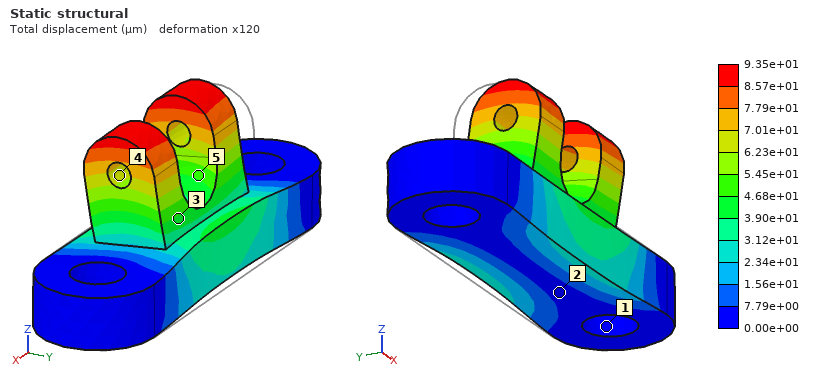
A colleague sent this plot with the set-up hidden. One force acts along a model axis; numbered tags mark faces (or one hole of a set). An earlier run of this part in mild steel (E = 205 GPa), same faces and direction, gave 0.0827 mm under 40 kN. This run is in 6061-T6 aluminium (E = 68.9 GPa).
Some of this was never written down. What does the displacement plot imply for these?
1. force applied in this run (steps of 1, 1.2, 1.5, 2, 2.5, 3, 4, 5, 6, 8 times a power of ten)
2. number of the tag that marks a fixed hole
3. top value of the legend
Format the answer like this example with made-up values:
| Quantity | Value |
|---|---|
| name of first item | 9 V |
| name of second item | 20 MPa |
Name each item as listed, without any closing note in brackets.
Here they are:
| Quantity | Value |
|---|---|
| force applied in this run | 15 kN |
| number of the tag that marks a fixed hole | 1 |
| top value of the legend | 9.35e+01 µm |
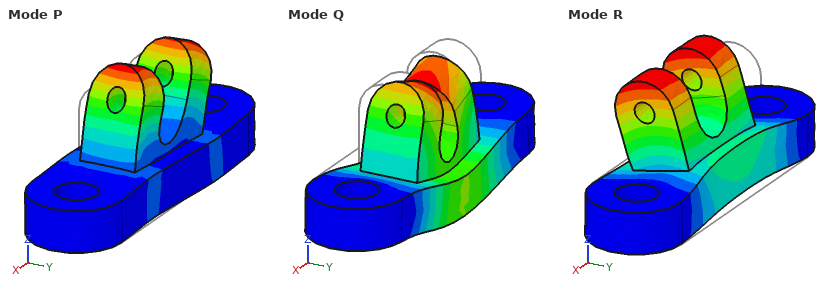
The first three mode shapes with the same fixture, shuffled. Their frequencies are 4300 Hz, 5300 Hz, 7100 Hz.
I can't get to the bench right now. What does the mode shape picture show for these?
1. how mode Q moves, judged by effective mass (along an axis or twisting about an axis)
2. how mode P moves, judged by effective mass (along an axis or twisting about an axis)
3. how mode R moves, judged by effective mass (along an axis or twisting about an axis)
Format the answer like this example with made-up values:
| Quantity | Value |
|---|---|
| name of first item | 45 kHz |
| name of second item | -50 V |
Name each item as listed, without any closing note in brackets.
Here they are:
| Quantity | Value |
|---|---|
| how mode Q moves, judged by effective mass | along Z |
| how mode P moves, judged by effective mass | along X |
| how mode R moves, judged by effective mass | along Y |
